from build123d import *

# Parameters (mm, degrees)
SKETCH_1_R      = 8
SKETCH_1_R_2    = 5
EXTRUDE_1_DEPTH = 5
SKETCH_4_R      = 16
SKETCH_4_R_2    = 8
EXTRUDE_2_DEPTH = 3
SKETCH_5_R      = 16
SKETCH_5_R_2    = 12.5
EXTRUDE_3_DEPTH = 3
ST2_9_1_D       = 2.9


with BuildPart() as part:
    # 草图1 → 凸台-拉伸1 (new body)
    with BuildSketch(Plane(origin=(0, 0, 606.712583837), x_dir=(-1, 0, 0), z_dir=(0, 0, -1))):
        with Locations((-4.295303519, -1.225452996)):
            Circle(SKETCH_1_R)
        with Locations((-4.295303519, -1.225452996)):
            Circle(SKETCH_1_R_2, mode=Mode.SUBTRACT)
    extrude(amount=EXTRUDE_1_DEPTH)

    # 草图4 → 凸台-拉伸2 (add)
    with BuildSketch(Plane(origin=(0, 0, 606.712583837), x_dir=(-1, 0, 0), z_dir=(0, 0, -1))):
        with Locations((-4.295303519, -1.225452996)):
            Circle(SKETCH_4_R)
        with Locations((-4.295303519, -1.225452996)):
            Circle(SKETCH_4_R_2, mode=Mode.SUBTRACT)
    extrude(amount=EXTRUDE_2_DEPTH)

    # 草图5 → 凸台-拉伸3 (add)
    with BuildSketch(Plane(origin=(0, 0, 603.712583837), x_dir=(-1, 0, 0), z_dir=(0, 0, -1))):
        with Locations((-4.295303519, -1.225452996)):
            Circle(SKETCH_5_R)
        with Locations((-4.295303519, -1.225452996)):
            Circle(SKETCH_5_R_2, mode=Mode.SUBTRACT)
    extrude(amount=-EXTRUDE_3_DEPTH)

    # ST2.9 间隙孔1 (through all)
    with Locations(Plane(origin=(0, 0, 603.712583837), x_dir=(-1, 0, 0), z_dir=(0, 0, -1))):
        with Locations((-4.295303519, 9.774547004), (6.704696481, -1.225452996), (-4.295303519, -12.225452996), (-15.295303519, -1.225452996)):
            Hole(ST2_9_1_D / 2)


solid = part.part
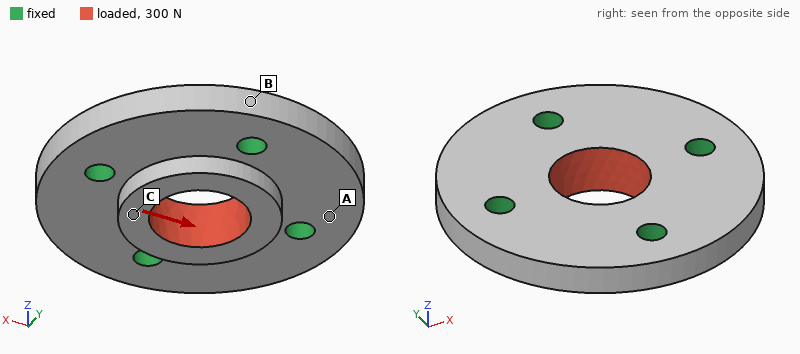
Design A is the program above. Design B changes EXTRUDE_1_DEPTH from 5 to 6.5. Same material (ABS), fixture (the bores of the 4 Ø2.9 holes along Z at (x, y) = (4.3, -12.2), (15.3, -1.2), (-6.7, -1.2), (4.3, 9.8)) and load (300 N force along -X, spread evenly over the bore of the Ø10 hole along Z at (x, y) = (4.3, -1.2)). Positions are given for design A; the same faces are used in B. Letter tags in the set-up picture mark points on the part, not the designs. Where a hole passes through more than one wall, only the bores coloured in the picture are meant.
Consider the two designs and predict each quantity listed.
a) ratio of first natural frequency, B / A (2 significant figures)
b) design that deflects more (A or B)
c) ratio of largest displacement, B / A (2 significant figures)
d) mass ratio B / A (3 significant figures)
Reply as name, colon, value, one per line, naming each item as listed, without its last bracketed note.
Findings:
ratio of first natural frequency, B / A: 1.0
design that deflects more: B
ratio of largest displacement, B / A: 1.3
mass ratio B / A: 1.08
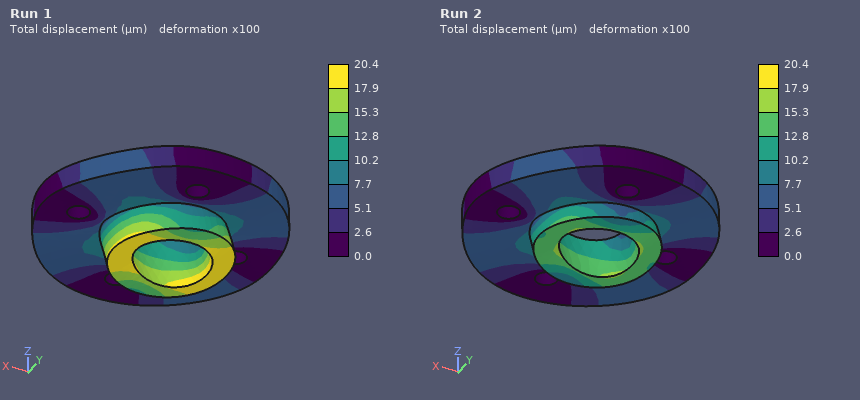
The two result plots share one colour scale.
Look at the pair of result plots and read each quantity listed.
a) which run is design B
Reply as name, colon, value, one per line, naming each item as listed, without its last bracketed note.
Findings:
which run is design B: Run 1
